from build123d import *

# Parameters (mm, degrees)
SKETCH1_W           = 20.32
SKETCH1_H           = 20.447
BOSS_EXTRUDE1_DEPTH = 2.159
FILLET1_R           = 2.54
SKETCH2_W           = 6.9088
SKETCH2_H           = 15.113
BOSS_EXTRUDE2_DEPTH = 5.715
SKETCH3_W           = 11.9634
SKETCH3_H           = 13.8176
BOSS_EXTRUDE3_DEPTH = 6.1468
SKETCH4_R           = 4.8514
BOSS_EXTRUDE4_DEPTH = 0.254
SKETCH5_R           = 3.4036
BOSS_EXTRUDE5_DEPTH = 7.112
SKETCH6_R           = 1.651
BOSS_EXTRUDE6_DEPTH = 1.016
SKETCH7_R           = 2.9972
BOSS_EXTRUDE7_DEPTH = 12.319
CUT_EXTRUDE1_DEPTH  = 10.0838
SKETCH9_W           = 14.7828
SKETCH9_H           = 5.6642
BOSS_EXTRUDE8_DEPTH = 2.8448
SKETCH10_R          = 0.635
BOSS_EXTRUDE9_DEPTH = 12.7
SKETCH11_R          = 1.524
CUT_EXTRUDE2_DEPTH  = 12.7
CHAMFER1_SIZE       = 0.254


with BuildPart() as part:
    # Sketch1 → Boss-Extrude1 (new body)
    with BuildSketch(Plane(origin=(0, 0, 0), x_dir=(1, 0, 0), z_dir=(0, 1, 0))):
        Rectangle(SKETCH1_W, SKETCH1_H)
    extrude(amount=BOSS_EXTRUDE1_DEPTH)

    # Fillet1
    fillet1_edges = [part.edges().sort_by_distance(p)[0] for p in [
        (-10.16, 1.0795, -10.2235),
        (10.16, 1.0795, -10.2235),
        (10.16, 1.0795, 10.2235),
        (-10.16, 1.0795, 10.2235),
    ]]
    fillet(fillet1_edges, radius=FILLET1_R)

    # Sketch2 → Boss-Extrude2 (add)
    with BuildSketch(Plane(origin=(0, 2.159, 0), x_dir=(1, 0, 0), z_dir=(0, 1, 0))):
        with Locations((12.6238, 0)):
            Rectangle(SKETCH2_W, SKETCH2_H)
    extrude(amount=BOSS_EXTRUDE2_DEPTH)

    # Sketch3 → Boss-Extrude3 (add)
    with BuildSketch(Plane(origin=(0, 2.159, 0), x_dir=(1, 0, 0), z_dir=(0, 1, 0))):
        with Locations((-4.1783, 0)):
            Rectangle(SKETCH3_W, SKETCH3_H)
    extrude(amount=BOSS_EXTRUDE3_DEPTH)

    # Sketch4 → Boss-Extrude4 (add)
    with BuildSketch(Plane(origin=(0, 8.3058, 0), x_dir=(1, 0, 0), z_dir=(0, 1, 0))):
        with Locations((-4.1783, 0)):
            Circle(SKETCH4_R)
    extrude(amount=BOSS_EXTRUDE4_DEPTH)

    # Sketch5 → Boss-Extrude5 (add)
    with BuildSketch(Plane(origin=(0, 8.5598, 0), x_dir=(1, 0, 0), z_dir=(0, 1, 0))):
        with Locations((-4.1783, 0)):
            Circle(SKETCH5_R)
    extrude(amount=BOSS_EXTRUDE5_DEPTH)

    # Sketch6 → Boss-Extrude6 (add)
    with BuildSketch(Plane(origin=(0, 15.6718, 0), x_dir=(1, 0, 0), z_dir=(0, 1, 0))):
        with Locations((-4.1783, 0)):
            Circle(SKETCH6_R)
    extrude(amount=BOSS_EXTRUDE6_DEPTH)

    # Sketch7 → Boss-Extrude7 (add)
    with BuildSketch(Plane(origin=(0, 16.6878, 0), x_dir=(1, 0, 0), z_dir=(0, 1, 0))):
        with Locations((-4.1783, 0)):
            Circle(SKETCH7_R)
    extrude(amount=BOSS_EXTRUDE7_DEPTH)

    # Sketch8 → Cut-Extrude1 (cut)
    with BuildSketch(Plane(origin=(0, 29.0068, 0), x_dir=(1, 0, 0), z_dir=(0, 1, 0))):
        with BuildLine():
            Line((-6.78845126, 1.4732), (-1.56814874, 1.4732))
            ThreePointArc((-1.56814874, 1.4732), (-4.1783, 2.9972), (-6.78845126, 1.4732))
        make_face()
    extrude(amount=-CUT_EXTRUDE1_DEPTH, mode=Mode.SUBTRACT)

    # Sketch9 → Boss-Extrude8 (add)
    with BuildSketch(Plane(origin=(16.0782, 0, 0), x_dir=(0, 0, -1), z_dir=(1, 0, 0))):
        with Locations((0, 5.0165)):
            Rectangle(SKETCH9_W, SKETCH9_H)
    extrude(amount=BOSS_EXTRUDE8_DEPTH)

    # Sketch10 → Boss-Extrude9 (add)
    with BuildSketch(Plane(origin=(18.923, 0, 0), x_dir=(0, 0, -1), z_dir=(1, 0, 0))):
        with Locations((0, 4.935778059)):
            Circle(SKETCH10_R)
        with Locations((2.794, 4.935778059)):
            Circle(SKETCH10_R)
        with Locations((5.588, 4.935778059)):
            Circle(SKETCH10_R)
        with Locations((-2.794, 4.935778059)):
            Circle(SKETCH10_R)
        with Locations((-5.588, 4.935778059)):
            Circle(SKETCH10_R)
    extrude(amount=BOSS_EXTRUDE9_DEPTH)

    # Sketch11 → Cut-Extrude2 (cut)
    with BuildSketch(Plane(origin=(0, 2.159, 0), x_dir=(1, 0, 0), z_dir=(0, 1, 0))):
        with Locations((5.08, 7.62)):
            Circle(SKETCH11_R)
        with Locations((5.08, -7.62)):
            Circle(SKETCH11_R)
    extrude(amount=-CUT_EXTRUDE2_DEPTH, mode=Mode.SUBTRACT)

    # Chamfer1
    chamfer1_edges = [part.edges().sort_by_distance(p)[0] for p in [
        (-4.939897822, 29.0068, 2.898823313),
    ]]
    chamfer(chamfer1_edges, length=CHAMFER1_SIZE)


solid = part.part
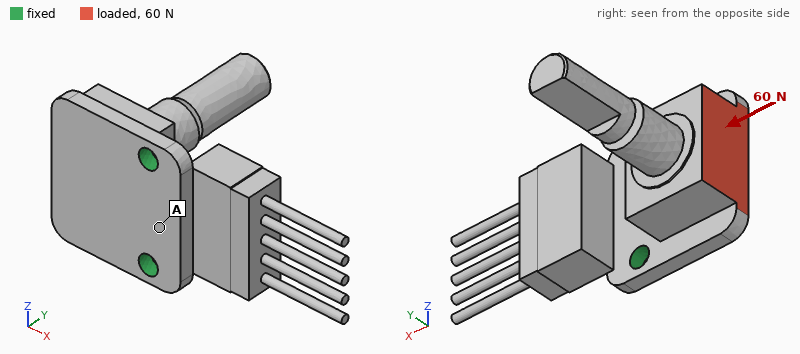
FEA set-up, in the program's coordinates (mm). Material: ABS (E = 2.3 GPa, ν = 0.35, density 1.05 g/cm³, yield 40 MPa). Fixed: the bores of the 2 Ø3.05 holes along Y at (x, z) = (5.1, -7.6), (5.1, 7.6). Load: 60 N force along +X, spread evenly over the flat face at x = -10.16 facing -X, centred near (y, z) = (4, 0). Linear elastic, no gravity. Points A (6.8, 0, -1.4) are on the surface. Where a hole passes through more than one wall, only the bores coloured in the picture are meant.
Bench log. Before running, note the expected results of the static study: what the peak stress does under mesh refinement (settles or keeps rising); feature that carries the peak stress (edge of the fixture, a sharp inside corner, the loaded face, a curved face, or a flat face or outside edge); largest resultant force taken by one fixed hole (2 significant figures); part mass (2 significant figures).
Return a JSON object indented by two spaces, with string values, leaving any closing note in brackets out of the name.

{
  "what the peak stress does under mesh refinement": "keeps rising",
  "feature that carries the peak stress": "edge of the fixture",
  "largest resultant force taken by one fixed hole": "31 N",
  "part mass": "3.5 g"
}
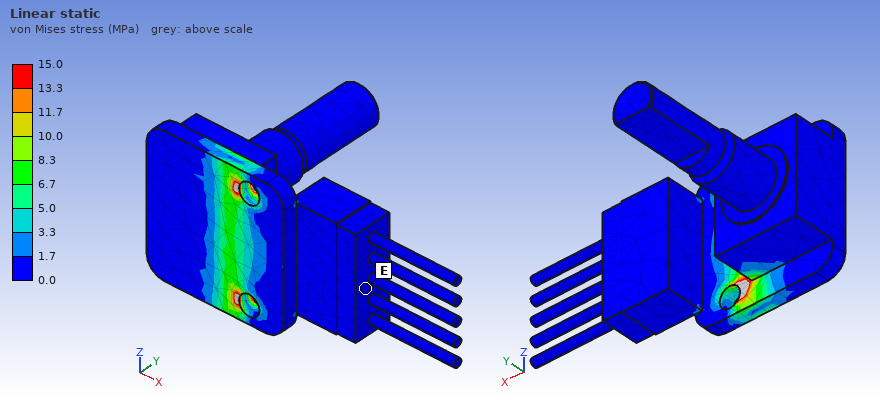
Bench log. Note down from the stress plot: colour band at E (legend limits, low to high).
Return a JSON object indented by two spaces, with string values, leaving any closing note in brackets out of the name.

{
  "colour band at E": "0.0 to 1.7 MPa"
}
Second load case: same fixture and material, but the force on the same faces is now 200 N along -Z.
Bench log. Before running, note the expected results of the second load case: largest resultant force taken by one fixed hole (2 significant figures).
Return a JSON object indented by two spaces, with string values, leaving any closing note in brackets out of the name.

{
  "largest resultant force taken by one fixed hole": "210 N"
}
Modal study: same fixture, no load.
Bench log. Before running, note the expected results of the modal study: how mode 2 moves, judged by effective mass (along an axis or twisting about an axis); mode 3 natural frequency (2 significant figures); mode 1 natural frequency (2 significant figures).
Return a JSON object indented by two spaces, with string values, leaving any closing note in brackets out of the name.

{
  "how mode 2 moves, judged by effective mass": "along Y",
  "mode 3 natural frequency": "1500 Hz",
  "mode 1 natural frequency": "850 Hz"
}
